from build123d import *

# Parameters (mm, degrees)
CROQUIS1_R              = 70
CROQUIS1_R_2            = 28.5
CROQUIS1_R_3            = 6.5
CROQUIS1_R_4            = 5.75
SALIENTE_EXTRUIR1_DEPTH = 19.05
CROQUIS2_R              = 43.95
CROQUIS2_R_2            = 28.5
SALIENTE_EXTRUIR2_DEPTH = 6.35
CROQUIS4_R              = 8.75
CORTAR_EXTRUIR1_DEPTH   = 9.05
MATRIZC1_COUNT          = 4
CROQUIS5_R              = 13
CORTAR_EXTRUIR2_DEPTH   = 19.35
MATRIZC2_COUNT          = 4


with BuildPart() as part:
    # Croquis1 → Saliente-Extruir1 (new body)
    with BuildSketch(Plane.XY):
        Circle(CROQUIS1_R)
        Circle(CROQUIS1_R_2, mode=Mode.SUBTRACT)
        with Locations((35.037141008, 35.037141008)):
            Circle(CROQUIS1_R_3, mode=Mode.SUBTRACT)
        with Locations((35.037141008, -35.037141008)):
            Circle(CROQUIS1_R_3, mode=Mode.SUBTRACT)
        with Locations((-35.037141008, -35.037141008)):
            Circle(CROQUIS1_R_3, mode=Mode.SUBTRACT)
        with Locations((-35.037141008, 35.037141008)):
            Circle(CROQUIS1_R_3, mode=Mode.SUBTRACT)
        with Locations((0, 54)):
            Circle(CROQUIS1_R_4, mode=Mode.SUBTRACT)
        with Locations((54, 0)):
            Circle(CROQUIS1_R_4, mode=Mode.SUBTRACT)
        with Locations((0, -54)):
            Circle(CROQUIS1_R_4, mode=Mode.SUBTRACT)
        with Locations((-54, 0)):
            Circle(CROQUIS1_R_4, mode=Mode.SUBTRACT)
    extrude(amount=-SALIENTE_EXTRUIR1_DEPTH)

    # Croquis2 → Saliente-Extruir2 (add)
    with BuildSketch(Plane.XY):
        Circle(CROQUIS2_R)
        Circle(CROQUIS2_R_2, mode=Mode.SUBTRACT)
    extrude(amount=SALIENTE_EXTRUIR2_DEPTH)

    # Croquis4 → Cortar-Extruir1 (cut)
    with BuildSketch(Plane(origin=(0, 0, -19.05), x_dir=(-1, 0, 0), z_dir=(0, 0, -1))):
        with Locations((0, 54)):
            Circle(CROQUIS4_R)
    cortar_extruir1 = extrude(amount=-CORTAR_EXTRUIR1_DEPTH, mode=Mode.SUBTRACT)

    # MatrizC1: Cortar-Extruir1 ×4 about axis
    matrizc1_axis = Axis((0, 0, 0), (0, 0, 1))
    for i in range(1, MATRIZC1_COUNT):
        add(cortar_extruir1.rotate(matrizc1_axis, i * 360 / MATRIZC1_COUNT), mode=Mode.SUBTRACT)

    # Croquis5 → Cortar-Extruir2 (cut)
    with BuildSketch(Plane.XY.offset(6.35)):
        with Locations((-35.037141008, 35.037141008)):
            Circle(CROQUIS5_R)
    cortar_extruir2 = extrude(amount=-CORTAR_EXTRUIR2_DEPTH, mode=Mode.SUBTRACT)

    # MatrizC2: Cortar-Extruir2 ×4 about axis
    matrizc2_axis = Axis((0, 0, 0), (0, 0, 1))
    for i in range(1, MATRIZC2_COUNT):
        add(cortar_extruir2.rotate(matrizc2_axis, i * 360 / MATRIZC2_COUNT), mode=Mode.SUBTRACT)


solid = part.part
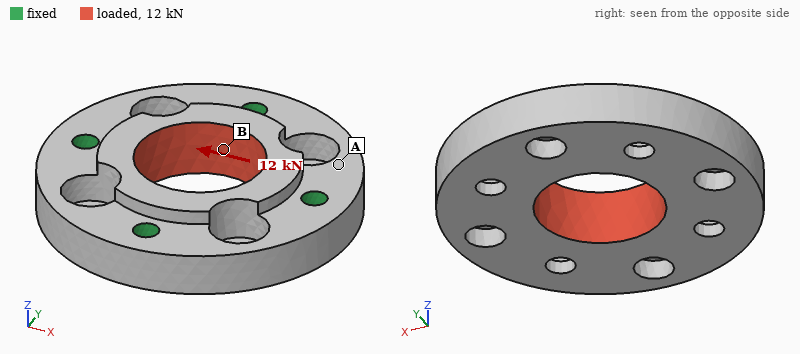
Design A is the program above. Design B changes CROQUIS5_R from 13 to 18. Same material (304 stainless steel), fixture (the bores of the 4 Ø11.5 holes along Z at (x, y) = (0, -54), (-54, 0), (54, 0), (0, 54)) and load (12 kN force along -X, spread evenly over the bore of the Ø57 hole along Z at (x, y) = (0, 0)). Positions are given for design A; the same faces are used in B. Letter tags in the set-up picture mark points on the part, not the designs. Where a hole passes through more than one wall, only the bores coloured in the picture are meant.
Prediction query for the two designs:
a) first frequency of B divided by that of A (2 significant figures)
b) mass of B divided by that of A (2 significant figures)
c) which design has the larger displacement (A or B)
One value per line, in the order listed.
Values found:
1.1
0.87
B
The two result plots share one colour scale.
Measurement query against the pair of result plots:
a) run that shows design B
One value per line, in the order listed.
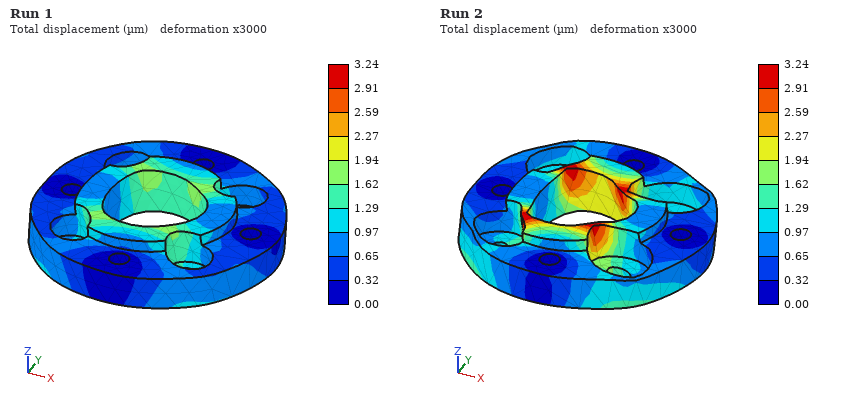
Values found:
Run 2
